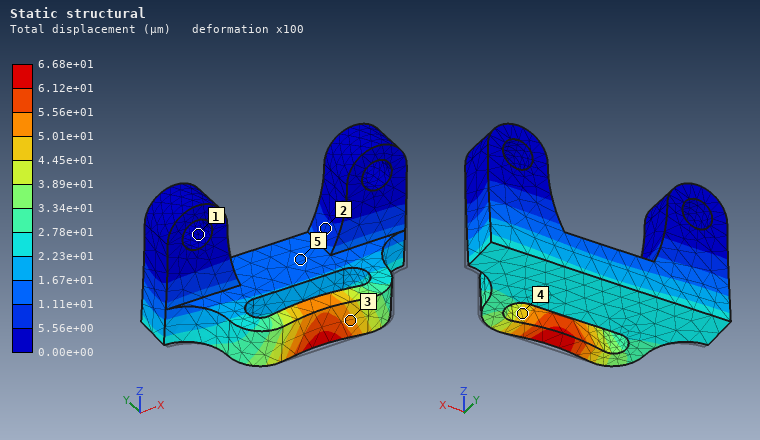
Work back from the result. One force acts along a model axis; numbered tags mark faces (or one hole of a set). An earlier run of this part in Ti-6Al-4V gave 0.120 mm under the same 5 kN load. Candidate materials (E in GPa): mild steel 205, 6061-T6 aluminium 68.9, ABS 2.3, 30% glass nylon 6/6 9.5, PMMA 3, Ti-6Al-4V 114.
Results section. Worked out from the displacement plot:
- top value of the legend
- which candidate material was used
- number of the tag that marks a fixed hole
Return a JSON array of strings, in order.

["6.68e+01 µm", "mild steel", "1"]
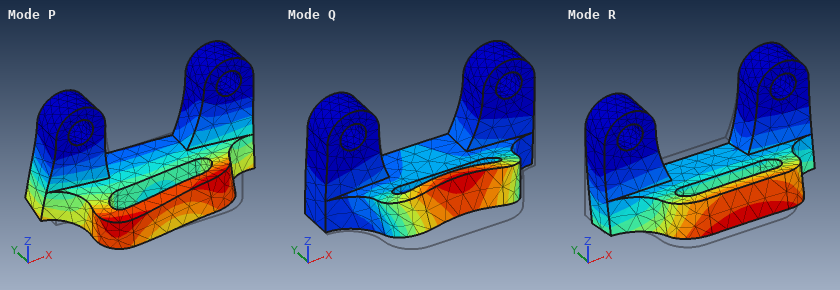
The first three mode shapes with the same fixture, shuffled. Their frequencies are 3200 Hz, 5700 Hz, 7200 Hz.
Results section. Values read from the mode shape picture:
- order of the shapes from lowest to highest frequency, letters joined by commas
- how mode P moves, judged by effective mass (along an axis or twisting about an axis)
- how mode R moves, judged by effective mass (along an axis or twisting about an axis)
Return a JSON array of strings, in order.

["R, P, Q", "along X", "along Y"]
